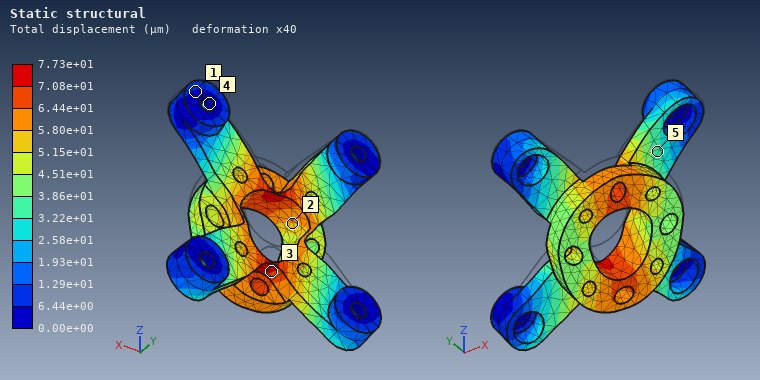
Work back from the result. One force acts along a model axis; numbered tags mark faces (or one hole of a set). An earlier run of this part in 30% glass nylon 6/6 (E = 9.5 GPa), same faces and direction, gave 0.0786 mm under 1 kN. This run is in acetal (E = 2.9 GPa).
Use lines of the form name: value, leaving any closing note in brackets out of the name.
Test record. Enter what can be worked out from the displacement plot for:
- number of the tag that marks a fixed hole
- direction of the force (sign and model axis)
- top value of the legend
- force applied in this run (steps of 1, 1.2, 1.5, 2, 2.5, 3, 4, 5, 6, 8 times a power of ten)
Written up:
number of the tag that marks a fixed hole: 4
direction of the force: -Z
top value of the legend: 7.73e+01 µm
force applied in this run: 300 N
